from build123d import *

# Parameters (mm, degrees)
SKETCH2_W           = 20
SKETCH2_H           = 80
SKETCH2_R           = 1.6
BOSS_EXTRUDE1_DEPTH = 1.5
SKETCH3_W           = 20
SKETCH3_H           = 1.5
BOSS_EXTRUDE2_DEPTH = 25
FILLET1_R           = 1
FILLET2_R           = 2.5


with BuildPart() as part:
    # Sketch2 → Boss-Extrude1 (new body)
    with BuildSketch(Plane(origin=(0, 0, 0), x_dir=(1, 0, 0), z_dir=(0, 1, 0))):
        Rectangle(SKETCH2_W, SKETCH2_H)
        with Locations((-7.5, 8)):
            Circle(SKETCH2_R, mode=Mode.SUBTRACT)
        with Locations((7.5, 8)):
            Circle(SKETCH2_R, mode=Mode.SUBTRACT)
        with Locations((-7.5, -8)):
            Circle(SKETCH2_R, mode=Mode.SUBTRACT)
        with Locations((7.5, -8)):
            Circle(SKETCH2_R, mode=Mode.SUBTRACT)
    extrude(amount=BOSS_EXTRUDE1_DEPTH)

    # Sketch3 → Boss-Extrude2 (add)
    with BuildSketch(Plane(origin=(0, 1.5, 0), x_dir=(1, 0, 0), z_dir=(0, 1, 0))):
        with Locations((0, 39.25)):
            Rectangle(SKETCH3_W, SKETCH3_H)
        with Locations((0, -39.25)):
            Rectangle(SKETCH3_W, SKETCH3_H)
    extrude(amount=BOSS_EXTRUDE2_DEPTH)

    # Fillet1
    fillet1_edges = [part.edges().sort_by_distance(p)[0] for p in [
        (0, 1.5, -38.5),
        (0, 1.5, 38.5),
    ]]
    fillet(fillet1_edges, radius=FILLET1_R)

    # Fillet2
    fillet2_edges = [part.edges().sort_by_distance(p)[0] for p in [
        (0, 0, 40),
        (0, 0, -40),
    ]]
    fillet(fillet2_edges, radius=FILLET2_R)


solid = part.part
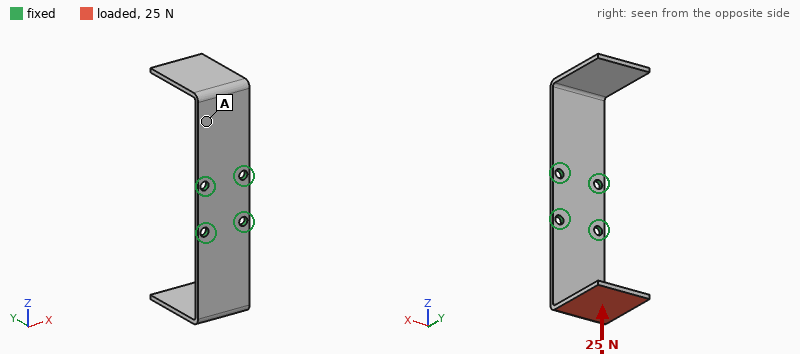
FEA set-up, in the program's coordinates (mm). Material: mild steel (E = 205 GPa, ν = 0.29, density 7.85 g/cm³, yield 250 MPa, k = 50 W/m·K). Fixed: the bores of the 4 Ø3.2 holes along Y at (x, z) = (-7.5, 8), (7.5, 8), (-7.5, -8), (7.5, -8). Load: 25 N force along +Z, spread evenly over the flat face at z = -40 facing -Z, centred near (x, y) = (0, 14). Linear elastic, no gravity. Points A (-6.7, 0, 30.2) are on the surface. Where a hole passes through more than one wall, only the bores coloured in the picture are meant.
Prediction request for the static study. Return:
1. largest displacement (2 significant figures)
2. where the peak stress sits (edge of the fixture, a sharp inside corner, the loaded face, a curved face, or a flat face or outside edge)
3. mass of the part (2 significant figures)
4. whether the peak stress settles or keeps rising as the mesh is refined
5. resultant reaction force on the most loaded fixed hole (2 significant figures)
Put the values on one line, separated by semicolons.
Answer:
0.31 mm; edge of the fixture; 30 g; keeps rising; 12 N
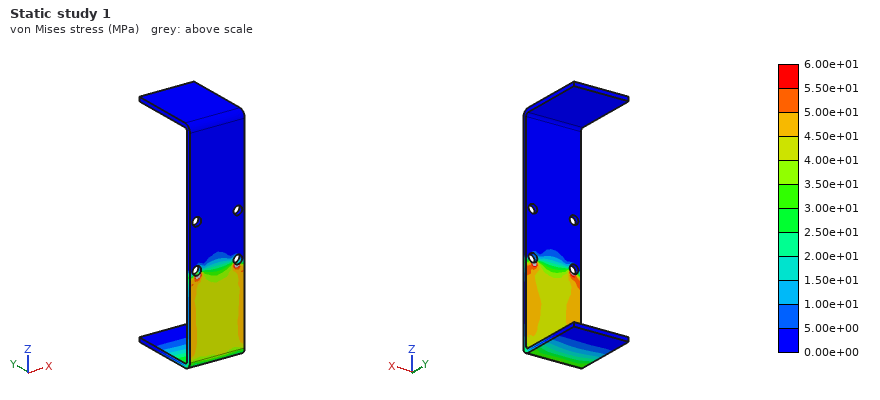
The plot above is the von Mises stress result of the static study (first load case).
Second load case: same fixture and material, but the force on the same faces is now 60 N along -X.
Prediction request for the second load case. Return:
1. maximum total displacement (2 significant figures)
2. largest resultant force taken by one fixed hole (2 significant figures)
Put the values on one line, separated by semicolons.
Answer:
0.31 mm; 130 N
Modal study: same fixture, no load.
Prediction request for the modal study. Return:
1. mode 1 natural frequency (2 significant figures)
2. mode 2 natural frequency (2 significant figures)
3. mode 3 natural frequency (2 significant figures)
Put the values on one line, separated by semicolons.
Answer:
520 Hz; 520 Hz; 1100 Hz
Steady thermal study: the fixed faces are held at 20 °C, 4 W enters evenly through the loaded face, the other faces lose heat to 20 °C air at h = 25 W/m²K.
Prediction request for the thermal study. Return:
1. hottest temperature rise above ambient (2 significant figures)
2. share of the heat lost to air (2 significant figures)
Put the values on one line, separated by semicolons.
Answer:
75 K; 46 %
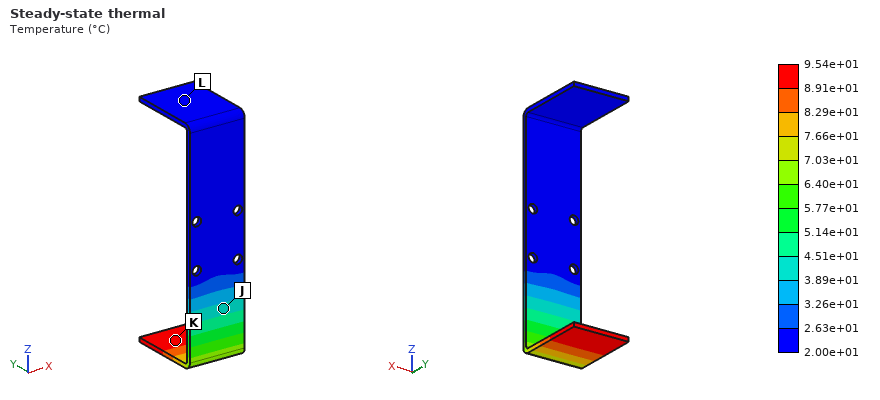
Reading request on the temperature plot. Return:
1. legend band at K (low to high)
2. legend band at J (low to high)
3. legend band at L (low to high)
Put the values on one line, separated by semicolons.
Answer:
8.91e+01 to 9.54e+01 °C; 3.89e+01 to 4.51e+01 °C; 2.00e+01 to 2.63e+01 °C
